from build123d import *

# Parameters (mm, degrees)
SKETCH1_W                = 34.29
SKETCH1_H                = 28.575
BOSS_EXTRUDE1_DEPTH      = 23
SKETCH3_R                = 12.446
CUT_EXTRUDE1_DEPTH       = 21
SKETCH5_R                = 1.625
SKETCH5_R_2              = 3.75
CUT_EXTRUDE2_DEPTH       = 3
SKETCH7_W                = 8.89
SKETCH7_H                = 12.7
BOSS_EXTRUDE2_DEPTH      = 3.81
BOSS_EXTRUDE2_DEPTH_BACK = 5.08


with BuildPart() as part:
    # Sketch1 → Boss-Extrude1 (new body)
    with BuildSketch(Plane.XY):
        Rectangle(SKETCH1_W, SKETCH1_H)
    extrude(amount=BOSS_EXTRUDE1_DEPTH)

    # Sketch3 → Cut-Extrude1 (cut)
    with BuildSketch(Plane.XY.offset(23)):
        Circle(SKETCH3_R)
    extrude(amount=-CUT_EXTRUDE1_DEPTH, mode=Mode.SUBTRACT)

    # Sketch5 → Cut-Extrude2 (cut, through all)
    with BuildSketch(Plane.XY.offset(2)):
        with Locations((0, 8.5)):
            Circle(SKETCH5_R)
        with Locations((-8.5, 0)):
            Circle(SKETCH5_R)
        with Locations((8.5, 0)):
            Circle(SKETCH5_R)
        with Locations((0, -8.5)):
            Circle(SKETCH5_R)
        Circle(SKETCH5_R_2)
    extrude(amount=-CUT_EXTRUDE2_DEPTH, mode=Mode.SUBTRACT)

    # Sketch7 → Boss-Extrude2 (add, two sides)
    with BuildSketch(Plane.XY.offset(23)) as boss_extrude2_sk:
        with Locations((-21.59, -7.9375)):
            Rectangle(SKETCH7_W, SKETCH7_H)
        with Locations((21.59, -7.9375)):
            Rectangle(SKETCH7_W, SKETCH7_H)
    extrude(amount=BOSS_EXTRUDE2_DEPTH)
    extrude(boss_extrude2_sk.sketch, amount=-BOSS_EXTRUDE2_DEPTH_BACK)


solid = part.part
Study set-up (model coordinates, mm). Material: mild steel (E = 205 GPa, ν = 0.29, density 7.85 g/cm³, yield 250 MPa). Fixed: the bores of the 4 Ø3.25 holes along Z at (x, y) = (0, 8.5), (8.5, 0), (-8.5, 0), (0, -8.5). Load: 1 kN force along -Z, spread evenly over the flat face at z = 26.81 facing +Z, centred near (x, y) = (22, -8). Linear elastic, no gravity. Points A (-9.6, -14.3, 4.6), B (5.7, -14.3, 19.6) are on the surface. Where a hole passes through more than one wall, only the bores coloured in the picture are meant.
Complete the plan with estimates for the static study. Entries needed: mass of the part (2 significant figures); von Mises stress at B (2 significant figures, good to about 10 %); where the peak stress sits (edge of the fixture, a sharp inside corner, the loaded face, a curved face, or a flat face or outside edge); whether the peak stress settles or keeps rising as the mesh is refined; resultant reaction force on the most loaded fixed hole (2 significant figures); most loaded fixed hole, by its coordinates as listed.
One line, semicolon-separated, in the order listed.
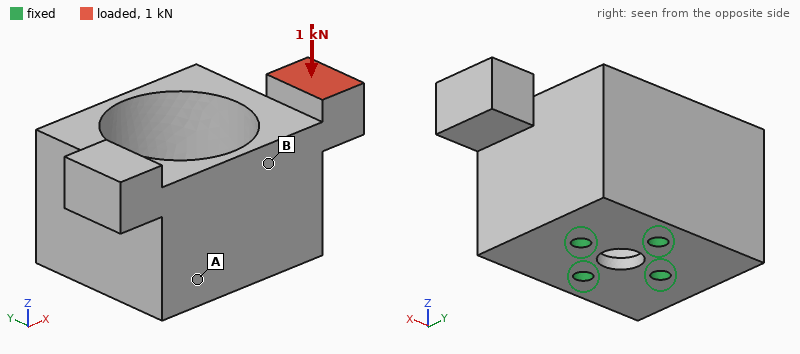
110 g; 33 MPa; edge of the fixture; keeps rising; 1.3 kN; (8.5, 0)
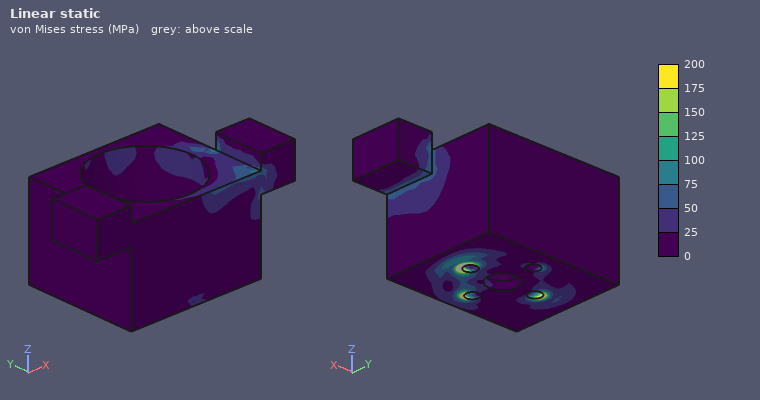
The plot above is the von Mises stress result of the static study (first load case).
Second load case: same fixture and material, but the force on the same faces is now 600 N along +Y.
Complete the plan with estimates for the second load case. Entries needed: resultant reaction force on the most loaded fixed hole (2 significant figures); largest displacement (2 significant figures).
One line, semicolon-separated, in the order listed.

760 N; 25 µm
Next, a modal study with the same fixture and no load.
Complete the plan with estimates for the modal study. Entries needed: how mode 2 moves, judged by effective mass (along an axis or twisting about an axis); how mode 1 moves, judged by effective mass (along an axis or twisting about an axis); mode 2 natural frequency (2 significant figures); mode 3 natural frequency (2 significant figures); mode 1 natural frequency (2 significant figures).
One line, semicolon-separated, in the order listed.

along Y; along X; 4800 Hz; 9700 Hz; 4300 Hz
